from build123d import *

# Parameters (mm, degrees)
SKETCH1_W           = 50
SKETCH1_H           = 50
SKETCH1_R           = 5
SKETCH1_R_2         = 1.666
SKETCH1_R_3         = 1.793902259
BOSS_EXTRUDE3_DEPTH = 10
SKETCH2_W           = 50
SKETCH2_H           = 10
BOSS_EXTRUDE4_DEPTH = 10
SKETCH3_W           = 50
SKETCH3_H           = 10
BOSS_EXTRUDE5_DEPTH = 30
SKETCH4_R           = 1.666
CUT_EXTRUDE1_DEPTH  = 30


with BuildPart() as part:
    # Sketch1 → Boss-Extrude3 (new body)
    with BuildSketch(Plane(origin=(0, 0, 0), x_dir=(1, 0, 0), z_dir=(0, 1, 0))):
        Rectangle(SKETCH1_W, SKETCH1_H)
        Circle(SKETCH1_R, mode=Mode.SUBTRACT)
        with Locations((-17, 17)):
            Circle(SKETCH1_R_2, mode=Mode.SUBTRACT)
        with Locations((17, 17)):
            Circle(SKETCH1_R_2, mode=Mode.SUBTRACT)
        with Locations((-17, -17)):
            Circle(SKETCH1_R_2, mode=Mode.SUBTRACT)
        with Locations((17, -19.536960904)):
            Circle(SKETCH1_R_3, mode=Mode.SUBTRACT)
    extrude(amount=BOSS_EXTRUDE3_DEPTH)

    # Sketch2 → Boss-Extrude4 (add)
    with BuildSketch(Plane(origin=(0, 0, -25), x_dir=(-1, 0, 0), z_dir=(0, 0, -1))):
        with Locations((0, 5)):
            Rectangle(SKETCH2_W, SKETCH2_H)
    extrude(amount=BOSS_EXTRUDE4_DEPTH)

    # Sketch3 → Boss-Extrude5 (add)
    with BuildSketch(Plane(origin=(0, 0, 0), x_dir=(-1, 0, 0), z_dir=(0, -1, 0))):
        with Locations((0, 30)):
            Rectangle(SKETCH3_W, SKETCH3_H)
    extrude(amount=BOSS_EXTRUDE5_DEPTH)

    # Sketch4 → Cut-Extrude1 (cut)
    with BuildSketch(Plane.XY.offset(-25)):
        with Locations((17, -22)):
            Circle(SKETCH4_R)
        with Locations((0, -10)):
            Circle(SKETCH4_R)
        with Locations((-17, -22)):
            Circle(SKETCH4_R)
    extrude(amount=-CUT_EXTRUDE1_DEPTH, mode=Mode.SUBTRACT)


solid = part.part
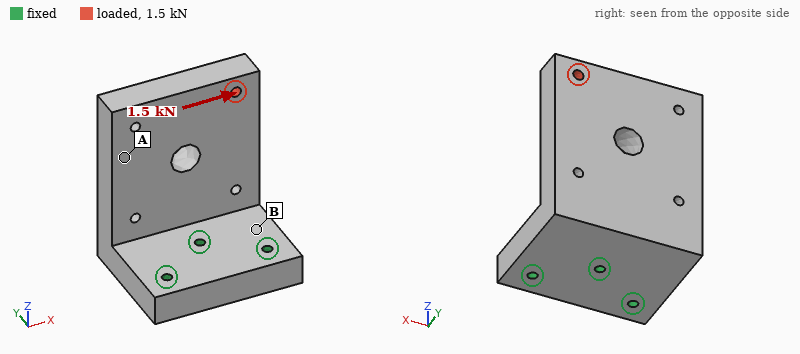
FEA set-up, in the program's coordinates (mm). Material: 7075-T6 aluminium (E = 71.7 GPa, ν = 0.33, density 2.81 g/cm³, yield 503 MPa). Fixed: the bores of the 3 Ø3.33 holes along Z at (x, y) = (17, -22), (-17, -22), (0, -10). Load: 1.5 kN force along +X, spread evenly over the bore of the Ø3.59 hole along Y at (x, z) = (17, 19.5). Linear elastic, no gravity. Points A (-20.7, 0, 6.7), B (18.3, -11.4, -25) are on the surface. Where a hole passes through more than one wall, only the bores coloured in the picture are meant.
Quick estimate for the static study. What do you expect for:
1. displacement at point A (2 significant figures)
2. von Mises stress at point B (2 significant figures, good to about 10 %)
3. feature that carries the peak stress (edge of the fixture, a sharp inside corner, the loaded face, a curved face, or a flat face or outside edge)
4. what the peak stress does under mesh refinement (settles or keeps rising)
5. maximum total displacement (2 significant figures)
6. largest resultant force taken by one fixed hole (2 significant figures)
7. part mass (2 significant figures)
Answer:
0.11 mm
40 MPa
edge of the fixture
keeps rising
0.15 mm
1.6 kN
120 g
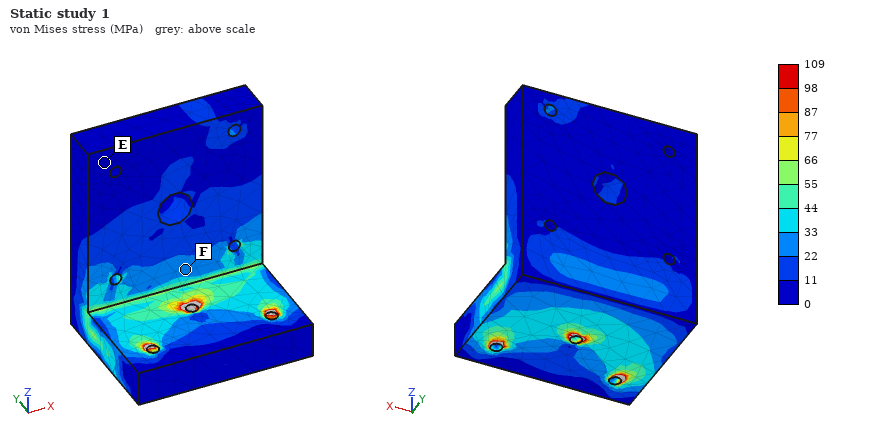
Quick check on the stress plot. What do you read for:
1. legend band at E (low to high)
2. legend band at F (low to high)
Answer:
0 to 11 MPa
22 to 33 MPa
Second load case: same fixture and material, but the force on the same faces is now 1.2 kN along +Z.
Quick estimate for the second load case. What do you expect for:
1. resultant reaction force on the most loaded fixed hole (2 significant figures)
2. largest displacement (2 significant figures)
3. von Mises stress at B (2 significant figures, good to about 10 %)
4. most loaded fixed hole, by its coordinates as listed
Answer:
1.4 kN
71 µm
20 MPa
(0, -10)
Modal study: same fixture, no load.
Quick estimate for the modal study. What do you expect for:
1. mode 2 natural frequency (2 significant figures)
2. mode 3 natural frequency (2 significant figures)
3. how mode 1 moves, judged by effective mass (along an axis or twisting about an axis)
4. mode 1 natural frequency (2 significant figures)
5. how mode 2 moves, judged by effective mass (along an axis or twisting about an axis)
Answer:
2900 Hz
5800 Hz
along Y
1800 Hz
along X
